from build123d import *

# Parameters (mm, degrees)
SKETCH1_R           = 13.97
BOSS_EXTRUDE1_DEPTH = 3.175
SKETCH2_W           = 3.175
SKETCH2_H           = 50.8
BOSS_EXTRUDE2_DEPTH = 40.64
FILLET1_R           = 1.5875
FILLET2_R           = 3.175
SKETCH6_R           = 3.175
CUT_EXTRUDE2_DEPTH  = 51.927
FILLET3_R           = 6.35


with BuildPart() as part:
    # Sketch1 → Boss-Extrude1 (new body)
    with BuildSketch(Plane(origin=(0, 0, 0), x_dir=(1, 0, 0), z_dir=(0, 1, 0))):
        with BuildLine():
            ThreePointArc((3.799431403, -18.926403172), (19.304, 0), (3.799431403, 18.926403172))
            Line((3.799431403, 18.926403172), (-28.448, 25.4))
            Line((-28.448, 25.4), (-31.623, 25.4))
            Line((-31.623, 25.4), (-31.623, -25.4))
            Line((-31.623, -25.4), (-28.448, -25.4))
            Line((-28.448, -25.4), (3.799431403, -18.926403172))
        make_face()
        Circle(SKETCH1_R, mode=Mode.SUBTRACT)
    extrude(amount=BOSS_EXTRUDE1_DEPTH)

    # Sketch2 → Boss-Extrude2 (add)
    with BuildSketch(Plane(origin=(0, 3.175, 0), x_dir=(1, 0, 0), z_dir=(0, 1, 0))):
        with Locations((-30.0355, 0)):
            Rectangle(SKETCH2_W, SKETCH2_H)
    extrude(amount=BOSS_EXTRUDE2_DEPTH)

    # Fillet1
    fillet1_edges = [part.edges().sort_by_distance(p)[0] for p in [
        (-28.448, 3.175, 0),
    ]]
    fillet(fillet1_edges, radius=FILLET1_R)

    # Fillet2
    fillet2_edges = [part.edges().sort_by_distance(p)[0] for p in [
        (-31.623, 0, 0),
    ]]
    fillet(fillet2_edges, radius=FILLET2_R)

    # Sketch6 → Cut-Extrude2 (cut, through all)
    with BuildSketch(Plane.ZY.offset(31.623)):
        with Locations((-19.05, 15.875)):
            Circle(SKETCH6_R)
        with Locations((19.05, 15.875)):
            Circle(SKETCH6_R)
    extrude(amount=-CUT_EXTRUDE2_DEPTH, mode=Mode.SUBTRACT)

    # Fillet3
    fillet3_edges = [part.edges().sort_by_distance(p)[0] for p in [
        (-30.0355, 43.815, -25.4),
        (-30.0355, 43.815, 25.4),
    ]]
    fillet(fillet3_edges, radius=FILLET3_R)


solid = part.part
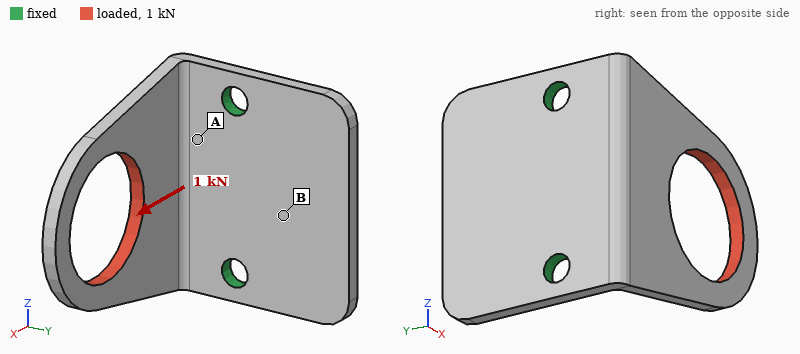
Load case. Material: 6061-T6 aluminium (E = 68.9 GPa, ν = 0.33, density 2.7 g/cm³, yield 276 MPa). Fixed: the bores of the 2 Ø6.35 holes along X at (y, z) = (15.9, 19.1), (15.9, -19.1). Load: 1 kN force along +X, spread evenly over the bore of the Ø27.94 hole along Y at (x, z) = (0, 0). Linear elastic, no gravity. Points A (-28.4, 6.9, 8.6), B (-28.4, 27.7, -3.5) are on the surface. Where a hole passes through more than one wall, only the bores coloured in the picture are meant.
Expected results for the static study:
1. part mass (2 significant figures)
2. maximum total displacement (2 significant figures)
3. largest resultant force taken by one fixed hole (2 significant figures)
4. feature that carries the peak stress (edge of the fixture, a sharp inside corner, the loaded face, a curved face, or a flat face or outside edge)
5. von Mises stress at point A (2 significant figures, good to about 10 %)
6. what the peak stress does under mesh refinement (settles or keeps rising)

29 g
0.46 mm
500 N
edge of the fixture
50 MPa
keeps rising
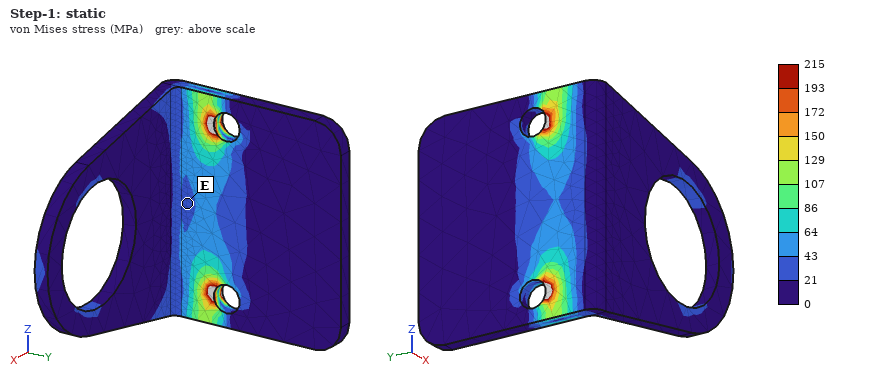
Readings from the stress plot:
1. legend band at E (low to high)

21 to 43 MPa
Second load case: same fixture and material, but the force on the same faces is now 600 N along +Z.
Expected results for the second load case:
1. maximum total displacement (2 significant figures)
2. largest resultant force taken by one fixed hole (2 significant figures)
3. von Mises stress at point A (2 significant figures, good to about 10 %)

0.19 mm
590 N
47 MPa
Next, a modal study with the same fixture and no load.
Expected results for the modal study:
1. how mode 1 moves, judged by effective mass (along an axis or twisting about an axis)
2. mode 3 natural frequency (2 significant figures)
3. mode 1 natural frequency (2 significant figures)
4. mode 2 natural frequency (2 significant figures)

along Y
3400 Hz
1200 Hz
3100 Hz
